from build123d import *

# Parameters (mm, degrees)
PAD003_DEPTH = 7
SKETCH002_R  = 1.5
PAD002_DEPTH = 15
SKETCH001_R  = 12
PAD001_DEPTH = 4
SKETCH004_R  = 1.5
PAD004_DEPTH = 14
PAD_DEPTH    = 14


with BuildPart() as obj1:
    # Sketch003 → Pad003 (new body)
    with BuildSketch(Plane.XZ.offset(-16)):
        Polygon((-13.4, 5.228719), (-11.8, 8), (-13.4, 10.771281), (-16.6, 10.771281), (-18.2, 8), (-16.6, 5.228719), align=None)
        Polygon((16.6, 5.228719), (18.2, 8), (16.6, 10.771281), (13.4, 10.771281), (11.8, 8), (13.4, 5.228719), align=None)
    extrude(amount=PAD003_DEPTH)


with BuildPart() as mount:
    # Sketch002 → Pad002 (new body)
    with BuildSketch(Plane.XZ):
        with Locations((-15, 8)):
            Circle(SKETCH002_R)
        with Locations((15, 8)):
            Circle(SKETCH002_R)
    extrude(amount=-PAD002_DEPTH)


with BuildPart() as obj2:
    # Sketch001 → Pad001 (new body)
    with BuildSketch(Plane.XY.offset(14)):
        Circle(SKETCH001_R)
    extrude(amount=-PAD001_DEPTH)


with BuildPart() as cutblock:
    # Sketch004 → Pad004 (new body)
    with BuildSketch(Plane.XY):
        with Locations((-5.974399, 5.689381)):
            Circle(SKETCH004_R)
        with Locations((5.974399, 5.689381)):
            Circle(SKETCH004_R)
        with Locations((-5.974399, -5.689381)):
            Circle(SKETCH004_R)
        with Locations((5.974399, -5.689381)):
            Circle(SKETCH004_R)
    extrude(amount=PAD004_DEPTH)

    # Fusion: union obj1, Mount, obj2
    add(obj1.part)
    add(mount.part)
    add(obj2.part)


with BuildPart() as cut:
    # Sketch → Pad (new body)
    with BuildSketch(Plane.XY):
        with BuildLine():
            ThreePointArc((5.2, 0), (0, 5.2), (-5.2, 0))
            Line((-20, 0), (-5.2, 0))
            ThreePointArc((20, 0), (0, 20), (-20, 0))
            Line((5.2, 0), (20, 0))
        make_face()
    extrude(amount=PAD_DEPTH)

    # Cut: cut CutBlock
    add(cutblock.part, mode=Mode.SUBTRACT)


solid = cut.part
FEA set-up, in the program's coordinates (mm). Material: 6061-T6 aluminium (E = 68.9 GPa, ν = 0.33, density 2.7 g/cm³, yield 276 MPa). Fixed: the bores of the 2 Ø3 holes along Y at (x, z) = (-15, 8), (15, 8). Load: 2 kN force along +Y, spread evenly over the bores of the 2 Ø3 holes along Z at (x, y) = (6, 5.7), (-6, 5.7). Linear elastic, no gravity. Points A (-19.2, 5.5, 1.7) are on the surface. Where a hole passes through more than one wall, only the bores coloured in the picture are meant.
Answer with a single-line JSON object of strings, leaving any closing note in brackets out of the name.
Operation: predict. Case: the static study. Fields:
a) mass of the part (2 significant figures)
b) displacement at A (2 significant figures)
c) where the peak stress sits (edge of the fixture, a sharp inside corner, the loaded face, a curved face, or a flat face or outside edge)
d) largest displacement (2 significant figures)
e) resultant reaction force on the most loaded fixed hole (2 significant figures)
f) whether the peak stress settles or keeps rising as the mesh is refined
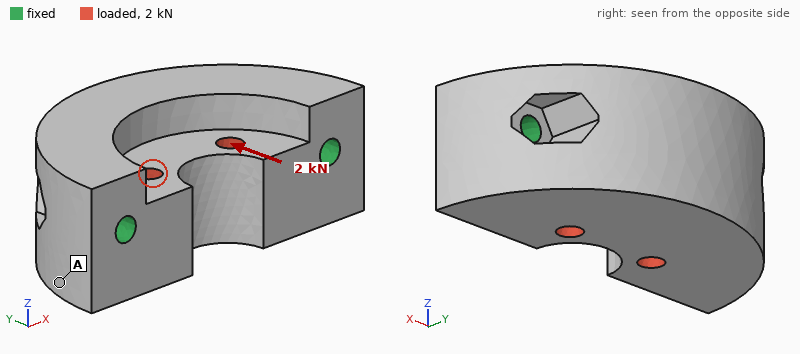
{"mass of the part": "19 g", "displacement at A": "1.4 µm", "where the peak stress sits": "edge of the fixture", "largest displacement": "7.7 µm", "resultant reaction force on the most loaded fixed hole": "1.1 kN", "whether the peak stress settles or keeps rising as the mesh is refined": "keeps rising"}
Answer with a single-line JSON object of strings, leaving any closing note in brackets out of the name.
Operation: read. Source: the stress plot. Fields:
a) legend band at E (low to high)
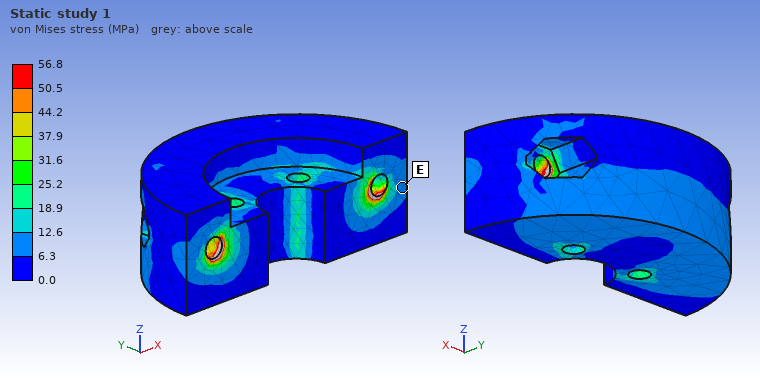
{"legend band at E": "6.3 to 12.6 MPa"}
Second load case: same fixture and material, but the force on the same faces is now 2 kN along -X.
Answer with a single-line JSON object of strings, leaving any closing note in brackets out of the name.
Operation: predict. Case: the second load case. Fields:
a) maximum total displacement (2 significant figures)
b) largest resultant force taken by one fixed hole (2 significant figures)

{"maximum total displacement": "3.1 µm", "largest resultant force taken by one fixed hole": "1.0 kN"}
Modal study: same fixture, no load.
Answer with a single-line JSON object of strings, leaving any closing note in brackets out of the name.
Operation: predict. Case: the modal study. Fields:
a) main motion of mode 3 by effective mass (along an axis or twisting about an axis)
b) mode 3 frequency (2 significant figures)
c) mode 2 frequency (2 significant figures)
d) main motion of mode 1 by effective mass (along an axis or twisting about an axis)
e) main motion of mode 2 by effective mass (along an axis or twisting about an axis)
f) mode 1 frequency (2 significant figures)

{"main motion of mode 3 by effective mass": "along X", "mode 3 frequency": "39 kHz", "mode 2 frequency": "34 kHz", "main motion of mode 1 by effective mass": "along Z", "main motion of mode 2 by effective mass": "along Y", "mode 1 frequency": "17 kHz"}
